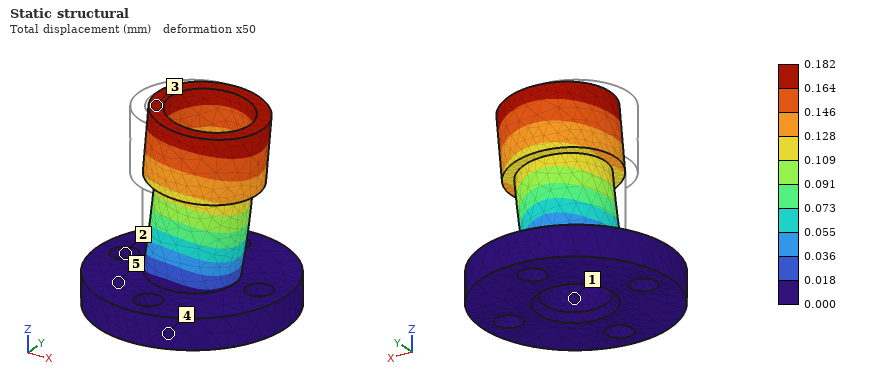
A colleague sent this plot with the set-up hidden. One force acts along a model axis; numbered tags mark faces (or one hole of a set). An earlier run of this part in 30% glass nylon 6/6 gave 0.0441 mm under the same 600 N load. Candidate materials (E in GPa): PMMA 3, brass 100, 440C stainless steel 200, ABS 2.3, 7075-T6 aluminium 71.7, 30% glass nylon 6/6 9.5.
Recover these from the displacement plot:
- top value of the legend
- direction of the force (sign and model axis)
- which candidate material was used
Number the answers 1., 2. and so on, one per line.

1. 0.182 mm
2. +X
3. ABS
